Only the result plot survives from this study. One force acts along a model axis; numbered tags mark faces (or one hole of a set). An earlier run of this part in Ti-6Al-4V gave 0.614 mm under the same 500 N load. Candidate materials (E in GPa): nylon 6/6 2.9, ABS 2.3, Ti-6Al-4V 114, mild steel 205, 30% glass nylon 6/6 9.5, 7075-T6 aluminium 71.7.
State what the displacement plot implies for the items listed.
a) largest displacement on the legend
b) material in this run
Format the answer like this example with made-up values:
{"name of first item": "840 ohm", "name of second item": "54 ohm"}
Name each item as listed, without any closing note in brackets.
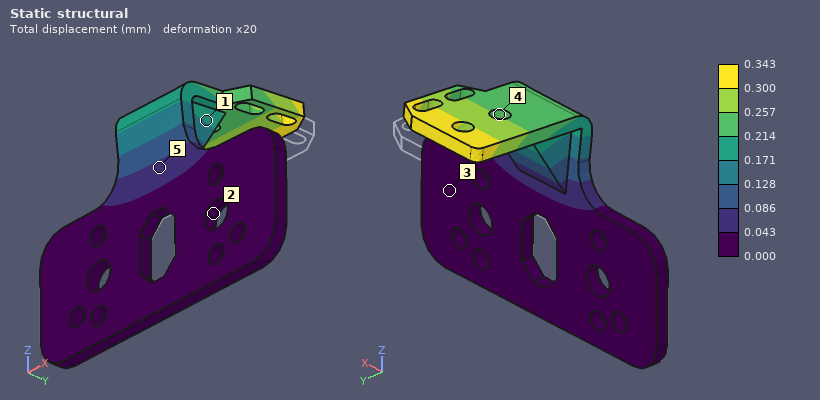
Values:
{"largest displacement on the legend": "0.343 mm", "material in this run": "mild steel"}
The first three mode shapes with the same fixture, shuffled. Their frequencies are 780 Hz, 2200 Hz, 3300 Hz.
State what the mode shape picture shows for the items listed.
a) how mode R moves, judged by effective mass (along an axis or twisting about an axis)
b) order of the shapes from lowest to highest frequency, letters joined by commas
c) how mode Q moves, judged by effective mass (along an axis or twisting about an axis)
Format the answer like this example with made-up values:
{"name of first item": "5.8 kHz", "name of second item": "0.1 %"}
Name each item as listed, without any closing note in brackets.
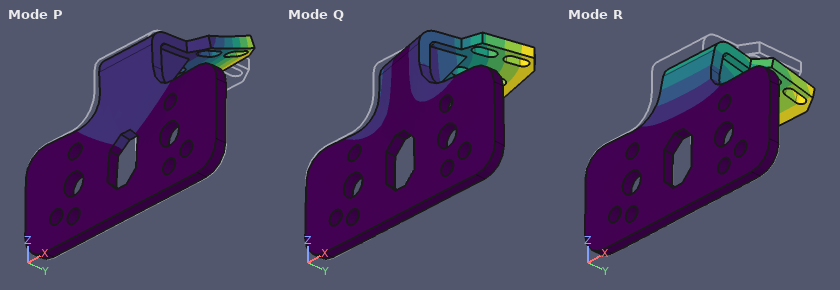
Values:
{"how mode R moves, judged by effective mass": "along Y", "order of the shapes from lowest to highest frequency, letters joined by commas": "R, Q, P", "how mode Q moves, judged by effective mass": "along X"}
